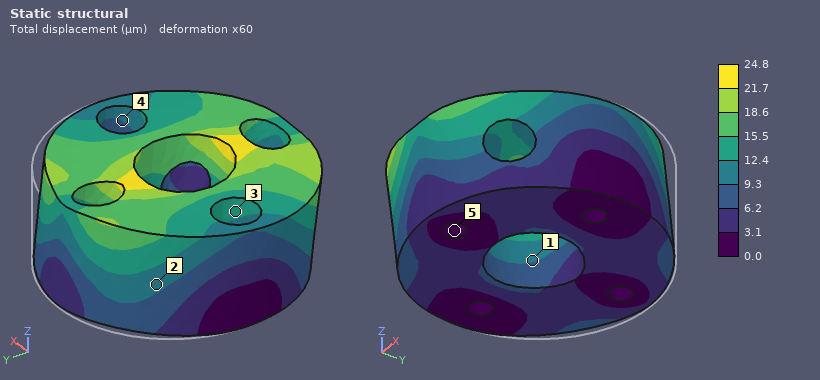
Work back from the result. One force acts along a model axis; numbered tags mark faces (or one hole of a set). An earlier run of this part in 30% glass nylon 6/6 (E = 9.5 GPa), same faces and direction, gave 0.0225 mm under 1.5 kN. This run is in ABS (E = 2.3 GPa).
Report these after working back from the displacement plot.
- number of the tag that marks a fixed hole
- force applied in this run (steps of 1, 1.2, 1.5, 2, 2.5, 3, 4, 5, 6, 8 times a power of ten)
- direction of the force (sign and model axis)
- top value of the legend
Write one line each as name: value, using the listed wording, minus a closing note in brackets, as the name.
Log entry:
number of the tag that marks a fixed hole: 5
force applied in this run: 400 N
direction of the force: -Y
top value of the legend: 24.8 µm
